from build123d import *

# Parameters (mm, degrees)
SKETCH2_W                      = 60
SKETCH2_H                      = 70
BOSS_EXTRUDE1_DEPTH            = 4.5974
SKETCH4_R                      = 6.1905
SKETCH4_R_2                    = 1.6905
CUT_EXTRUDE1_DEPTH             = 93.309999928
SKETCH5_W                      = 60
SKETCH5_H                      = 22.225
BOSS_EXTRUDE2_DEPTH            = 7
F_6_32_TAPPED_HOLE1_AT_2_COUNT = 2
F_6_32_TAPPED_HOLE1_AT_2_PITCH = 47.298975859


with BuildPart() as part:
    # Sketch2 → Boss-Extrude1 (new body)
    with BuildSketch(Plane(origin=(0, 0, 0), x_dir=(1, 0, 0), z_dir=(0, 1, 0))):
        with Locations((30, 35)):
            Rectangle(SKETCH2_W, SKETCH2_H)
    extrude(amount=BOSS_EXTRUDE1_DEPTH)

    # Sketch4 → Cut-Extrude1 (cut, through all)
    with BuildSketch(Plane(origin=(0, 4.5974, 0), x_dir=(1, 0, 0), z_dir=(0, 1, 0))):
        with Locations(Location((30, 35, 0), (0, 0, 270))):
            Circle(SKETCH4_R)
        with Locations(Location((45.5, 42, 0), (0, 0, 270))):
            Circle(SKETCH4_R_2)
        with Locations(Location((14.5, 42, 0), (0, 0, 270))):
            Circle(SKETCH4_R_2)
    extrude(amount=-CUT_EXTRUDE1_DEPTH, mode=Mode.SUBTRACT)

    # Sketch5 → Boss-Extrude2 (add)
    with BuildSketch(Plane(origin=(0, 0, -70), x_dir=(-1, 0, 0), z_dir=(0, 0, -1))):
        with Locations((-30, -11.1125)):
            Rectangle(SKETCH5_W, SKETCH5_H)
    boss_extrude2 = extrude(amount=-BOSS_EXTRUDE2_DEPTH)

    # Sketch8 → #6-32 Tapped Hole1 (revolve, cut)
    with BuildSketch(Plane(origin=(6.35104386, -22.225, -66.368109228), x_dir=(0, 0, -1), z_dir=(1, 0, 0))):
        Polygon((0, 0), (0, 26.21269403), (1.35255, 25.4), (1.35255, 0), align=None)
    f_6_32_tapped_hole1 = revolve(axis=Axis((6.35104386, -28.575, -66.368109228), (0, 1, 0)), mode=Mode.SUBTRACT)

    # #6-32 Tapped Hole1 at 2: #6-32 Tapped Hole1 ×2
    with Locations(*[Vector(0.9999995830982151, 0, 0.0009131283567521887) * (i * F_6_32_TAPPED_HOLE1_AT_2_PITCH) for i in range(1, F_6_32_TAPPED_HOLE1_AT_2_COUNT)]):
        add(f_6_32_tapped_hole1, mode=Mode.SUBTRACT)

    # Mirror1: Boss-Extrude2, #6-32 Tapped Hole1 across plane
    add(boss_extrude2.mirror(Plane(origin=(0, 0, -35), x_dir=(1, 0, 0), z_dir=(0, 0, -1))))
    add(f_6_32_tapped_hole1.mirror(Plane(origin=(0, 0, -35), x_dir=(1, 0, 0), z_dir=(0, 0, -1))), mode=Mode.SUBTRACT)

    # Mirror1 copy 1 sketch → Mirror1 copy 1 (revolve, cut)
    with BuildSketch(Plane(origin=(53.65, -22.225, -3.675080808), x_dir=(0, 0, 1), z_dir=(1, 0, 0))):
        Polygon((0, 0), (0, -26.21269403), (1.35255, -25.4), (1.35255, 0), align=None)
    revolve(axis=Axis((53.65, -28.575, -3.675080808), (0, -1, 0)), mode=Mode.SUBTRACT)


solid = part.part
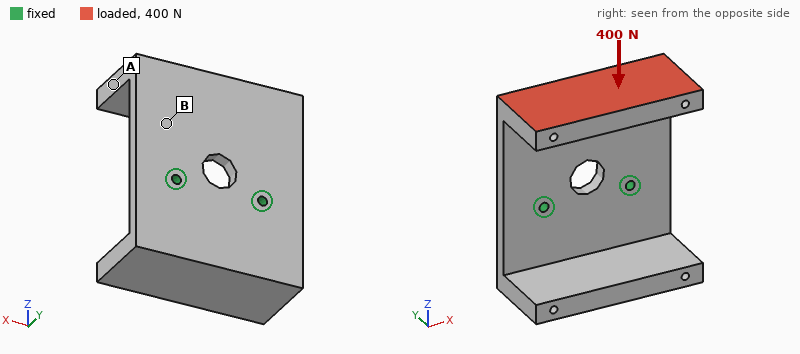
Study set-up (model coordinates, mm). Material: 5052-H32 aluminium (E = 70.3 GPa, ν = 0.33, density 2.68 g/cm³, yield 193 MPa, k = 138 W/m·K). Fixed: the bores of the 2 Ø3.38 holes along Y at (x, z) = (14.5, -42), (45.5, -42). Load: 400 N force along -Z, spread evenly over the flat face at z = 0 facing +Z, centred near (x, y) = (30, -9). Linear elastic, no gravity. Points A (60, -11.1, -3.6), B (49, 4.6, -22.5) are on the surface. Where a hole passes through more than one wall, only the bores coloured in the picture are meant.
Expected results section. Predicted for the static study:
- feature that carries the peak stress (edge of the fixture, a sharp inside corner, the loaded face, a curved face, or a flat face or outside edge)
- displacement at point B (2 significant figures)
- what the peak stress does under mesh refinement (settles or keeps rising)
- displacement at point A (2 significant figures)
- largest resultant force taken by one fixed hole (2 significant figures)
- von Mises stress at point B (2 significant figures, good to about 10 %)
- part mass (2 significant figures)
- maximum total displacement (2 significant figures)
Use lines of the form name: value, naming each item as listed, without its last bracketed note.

feature that carries the peak stress: edge of the fixture
displacement at point B: 0.034 mm
what the peak stress does under mesh refinement: keeps rising
displacement at point A: 0.13 mm
largest resultant force taken by one fixed hole: 200 N
von Mises stress at point B: 19 MPa
part mass: 98 g
maximum total displacement: 0.19 mm
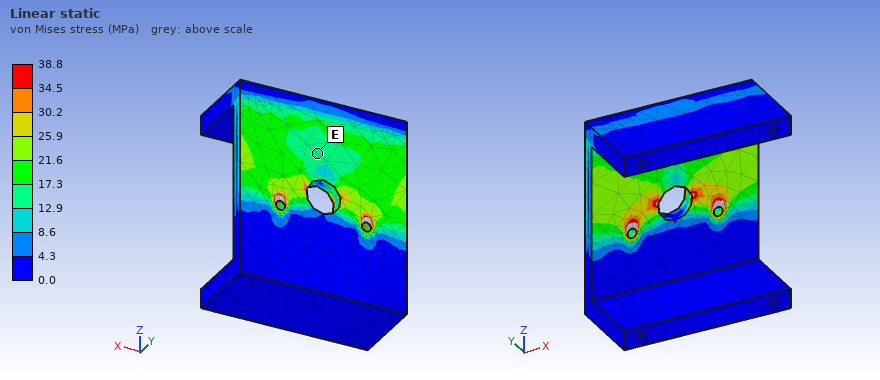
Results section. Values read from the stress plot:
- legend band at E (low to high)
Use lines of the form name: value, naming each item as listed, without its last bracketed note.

legend band at E: 12.9 to 17.3 MPa
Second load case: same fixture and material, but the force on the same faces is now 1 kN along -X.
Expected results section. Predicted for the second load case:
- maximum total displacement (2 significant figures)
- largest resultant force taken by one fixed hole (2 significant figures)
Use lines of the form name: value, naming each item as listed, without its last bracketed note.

maximum total displacement: 0.17 mm
largest resultant force taken by one fixed hole: 1.4 kN
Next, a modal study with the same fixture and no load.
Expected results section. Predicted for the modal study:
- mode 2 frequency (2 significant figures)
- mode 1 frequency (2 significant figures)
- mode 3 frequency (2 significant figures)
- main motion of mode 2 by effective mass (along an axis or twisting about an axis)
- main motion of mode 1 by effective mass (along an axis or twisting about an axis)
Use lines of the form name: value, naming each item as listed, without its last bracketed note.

mode 2 frequency: 1700 Hz
mode 1 frequency: 920 Hz
mode 3 frequency: 2000 Hz
main motion of mode 2 by effective mass: along Y
main motion of mode 1 by effective mass: along Y
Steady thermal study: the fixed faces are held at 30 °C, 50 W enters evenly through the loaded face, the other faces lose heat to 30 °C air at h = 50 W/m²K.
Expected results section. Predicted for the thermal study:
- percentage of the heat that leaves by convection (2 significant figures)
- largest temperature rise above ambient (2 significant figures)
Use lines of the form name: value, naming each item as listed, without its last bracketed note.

percentage of the heat that leaves by convection: 28 %
largest temperature rise above ambient: 54 K
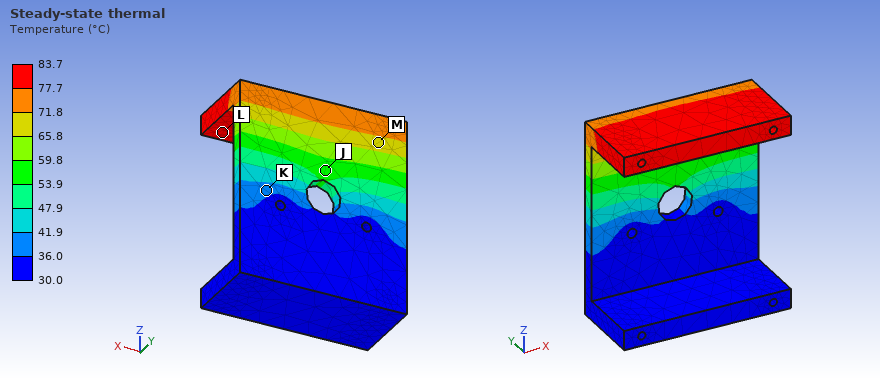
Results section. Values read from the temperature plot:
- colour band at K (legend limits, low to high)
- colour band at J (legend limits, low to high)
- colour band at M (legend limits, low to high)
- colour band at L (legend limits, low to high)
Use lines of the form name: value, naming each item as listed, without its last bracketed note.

colour band at K: 36.0 to 41.9 °C
colour band at J: 53.9 to 59.8 °C
colour band at M: 65.8 to 71.8 °C
colour band at L: 77.7 to 83.7 °C
